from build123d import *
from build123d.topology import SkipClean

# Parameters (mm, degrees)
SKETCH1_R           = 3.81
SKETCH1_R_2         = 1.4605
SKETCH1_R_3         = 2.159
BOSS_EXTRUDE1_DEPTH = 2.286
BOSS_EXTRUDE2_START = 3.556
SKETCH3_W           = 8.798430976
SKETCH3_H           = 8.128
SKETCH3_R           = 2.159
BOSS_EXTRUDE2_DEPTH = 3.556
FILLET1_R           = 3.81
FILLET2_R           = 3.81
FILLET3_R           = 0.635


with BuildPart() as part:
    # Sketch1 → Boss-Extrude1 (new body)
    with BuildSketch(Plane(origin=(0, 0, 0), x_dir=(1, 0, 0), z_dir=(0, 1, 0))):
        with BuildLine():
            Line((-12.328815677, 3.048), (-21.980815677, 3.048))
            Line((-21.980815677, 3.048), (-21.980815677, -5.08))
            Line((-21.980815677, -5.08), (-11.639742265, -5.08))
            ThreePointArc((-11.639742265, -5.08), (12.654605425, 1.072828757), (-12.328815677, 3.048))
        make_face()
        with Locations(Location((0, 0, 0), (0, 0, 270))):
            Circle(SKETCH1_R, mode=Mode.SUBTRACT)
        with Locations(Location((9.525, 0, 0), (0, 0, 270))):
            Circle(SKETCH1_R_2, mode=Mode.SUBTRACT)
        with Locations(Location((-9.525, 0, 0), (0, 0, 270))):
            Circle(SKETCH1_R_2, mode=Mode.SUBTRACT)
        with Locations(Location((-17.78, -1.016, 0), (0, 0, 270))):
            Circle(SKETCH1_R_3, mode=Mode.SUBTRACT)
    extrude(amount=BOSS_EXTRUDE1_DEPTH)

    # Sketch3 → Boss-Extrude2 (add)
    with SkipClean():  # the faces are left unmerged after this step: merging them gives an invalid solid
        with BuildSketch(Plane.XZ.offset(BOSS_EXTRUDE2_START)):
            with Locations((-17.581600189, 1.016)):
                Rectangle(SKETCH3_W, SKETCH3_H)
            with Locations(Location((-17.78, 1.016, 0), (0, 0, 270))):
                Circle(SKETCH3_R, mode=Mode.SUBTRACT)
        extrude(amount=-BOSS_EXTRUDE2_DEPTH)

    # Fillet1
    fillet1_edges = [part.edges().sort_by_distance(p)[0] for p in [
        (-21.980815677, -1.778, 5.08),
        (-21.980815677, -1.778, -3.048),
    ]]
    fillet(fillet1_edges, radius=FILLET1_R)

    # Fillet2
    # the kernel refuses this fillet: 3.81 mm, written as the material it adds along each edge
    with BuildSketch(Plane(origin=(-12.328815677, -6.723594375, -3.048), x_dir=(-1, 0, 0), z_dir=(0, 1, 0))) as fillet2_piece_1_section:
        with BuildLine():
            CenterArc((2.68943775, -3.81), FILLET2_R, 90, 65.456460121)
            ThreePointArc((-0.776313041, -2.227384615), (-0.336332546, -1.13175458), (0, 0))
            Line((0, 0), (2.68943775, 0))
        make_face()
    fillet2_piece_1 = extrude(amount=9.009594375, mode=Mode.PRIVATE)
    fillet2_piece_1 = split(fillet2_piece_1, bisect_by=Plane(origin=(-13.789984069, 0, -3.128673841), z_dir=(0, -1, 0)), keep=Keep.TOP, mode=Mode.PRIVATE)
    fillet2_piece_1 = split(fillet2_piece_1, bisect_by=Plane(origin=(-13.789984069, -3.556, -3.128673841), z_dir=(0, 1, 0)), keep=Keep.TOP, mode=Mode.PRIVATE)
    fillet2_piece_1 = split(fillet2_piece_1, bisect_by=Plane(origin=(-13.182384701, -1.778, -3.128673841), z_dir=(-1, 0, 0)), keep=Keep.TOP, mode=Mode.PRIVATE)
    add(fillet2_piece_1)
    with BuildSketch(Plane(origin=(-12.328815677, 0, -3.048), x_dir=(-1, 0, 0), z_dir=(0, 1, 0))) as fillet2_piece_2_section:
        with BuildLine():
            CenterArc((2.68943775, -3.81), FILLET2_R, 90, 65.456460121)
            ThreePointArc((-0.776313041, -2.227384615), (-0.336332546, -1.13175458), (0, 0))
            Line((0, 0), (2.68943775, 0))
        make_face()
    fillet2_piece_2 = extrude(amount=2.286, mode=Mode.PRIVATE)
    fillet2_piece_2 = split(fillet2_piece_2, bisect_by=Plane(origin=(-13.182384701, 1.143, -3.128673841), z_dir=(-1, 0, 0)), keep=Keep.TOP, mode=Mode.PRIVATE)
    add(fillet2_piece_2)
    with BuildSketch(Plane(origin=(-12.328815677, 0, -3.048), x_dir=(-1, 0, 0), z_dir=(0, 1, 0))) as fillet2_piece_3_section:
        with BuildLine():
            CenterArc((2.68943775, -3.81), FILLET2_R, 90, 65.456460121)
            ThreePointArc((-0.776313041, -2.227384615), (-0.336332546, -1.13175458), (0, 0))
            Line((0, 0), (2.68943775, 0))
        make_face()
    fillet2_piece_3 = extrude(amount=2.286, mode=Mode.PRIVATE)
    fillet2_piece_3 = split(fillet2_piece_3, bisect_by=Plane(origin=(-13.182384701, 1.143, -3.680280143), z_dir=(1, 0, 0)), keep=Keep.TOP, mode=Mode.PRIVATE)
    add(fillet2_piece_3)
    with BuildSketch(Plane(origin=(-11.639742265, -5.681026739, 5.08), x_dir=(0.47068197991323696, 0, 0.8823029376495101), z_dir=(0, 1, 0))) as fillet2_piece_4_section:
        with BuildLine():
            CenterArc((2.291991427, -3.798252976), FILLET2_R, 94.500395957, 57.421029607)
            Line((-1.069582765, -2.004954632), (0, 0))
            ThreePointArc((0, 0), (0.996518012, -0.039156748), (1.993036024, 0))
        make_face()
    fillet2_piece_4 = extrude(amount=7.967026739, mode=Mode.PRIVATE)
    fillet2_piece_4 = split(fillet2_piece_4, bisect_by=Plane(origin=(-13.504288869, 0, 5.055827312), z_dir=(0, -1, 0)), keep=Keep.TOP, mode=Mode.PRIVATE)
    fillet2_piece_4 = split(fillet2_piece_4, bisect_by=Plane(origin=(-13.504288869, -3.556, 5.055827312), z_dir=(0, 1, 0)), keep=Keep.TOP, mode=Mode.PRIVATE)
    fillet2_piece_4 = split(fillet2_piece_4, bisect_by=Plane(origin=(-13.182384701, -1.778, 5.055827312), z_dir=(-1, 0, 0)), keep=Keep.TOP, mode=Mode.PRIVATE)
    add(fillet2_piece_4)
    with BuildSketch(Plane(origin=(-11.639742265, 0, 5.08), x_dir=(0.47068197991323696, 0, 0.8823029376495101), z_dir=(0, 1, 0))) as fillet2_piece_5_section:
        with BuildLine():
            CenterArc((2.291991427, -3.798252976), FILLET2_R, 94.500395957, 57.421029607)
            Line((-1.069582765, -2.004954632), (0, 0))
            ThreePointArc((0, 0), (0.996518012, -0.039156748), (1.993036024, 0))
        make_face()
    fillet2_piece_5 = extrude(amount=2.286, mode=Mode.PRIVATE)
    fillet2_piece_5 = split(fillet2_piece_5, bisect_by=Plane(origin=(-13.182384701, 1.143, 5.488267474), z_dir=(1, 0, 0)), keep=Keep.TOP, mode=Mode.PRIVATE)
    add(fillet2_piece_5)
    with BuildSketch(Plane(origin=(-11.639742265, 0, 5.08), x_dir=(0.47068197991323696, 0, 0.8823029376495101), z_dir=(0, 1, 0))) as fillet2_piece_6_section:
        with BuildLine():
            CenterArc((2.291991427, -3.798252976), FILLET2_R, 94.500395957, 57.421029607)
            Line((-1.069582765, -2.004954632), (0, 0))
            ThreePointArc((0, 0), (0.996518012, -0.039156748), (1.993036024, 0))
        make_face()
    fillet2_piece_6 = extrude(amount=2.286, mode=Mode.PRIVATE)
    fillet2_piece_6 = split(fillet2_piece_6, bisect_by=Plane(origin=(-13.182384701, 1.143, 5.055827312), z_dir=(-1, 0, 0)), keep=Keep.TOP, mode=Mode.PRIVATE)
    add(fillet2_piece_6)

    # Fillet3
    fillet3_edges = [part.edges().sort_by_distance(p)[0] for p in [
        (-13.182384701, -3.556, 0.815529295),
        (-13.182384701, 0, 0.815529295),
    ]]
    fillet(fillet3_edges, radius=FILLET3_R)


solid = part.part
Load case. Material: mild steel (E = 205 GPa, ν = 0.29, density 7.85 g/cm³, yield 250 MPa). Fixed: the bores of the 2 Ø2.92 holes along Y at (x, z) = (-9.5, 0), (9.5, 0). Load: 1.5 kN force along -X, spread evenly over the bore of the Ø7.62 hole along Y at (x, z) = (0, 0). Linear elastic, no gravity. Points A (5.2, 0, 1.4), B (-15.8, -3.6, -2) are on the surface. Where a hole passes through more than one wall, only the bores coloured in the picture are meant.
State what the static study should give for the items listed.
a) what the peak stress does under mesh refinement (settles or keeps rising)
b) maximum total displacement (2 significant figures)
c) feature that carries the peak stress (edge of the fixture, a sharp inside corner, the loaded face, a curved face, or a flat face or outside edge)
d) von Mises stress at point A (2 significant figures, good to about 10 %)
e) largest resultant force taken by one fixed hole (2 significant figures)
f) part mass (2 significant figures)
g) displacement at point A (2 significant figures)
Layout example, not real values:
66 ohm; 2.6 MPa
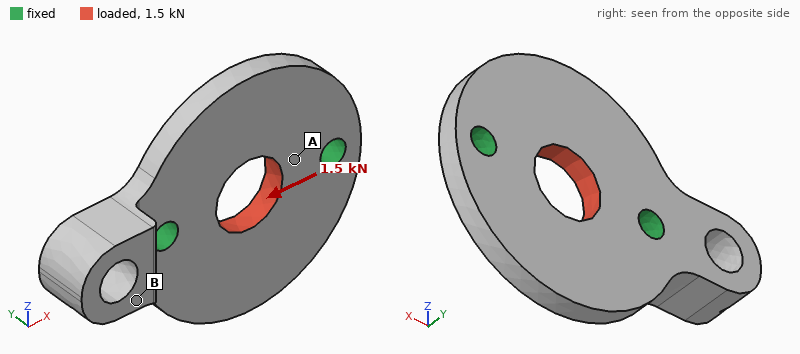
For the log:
keeps rising; 1.6 µm; edge of the fixture; 42 MPa; 770 N; 11 g; 0.78 µm
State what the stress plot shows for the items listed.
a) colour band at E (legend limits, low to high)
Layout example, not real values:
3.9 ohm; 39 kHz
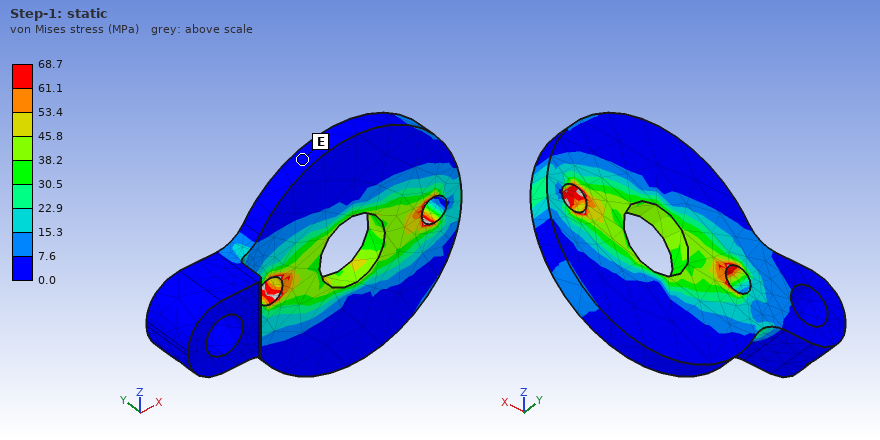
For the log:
0.0 to 7.6 MPa
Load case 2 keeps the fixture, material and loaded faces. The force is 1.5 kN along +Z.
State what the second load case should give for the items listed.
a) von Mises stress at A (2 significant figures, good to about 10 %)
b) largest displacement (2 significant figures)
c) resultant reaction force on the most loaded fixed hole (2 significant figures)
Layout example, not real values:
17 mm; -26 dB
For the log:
37 MPa; 2.2 µm; 750 N
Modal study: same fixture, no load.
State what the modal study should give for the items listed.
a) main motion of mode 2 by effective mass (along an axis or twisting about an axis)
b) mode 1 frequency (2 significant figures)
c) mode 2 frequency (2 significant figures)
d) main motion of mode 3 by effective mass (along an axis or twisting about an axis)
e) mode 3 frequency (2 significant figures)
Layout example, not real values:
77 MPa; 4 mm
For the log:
twisting about X; 11 kHz; 12 kHz; along Y; 14 kHz
